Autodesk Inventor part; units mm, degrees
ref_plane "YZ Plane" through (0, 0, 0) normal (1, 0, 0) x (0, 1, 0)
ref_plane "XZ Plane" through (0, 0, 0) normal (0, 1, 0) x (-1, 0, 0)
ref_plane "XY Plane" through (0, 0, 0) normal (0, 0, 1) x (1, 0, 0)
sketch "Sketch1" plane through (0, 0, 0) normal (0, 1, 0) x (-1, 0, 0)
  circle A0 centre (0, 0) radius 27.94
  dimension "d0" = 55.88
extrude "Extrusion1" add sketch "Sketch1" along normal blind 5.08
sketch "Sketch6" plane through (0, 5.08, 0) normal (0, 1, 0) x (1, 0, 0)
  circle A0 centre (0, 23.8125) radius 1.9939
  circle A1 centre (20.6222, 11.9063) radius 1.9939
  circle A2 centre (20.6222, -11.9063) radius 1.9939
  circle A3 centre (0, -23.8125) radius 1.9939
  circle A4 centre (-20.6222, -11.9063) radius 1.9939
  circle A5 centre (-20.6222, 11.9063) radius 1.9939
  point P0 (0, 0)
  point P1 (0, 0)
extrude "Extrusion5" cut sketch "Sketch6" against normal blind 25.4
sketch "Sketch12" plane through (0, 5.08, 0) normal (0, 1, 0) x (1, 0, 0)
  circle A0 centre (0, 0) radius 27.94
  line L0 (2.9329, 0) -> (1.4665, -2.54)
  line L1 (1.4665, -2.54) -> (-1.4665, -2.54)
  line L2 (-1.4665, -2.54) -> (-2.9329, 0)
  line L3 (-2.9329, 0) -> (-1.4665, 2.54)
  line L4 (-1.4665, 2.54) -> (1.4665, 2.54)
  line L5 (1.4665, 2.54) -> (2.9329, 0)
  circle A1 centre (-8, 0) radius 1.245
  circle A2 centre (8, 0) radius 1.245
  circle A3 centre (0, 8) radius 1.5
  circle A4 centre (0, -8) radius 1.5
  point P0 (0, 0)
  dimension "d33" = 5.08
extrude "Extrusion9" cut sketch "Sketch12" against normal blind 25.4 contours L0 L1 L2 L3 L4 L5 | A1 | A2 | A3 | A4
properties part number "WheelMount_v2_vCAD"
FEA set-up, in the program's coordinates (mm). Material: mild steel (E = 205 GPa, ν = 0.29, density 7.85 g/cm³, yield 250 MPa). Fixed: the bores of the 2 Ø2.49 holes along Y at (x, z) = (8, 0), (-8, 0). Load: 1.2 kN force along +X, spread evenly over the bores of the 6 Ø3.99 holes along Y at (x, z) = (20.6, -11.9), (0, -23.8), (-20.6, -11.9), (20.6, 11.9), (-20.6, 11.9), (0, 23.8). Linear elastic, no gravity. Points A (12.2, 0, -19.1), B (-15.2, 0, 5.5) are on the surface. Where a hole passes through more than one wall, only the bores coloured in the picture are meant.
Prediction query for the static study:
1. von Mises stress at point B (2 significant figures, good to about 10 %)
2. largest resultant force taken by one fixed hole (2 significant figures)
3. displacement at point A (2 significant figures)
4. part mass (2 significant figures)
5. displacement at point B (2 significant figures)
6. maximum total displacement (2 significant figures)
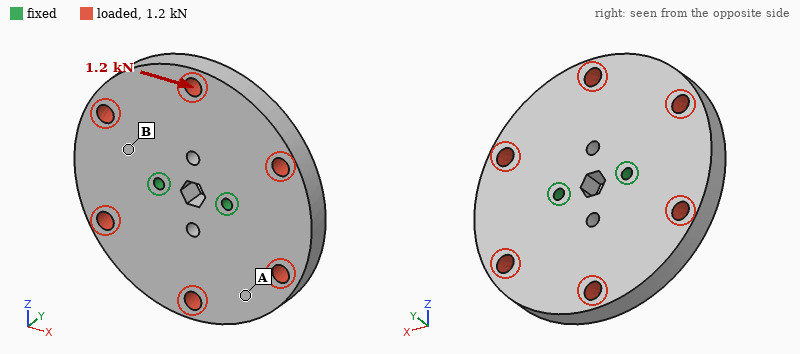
5.4 MPa
600 N
0.76 µm
93 g
0.40 µm
1.0 µm
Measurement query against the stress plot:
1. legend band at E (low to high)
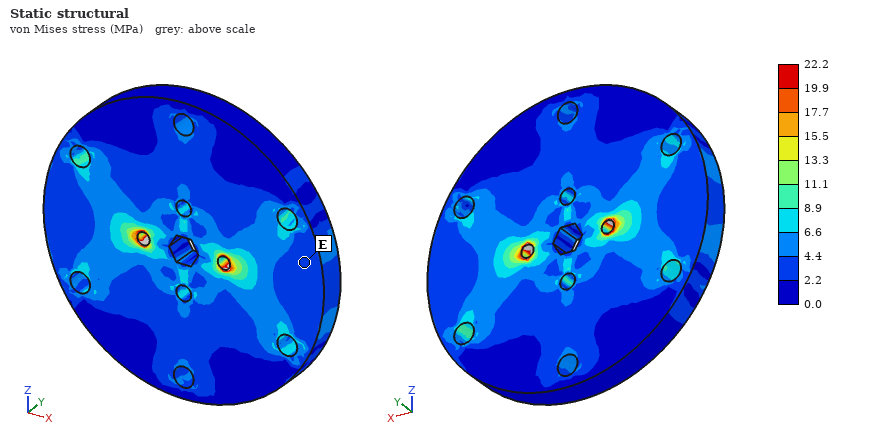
2.2 to 4.4 MPa
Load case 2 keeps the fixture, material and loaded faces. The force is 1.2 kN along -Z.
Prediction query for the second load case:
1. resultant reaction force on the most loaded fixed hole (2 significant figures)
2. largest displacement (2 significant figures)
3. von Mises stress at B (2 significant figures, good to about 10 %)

600 N
0.77 µm
3.7 MPa
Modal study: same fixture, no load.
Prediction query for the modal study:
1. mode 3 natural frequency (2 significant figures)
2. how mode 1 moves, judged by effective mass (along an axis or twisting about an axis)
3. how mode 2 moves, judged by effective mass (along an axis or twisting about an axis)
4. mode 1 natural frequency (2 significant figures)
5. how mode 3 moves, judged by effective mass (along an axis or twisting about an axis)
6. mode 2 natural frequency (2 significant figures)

8200 Hz
twisting about X
along Y
4700 Hz
twisting about Z
6700 Hz
